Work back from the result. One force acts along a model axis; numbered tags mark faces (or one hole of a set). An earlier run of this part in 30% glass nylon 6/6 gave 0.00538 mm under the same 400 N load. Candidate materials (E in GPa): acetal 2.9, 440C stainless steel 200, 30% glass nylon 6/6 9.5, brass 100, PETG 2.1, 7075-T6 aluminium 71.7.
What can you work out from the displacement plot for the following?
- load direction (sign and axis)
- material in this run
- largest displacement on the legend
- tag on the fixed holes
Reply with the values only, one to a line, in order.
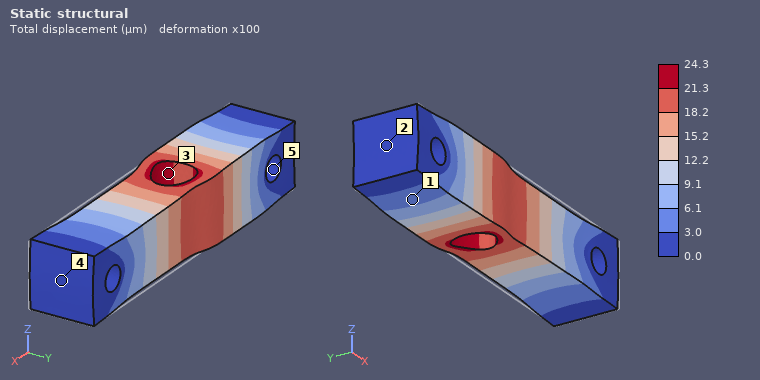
-X
PETG
24.3 µm
5
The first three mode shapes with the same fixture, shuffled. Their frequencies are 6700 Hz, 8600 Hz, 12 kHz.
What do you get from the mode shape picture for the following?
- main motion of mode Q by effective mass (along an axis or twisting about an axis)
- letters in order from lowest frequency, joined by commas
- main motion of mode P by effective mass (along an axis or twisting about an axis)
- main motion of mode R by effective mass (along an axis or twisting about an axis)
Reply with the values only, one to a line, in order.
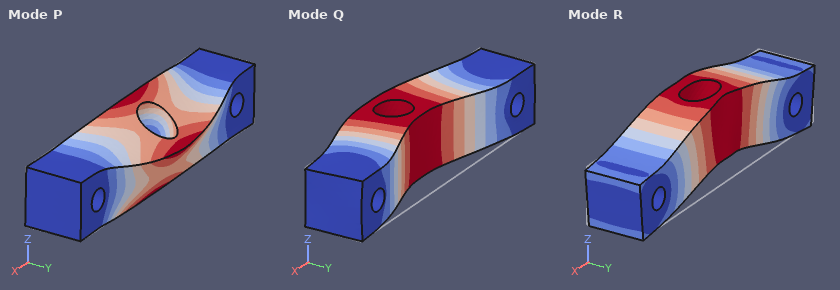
along Y
R, Q, P
twisting about X
along Z
